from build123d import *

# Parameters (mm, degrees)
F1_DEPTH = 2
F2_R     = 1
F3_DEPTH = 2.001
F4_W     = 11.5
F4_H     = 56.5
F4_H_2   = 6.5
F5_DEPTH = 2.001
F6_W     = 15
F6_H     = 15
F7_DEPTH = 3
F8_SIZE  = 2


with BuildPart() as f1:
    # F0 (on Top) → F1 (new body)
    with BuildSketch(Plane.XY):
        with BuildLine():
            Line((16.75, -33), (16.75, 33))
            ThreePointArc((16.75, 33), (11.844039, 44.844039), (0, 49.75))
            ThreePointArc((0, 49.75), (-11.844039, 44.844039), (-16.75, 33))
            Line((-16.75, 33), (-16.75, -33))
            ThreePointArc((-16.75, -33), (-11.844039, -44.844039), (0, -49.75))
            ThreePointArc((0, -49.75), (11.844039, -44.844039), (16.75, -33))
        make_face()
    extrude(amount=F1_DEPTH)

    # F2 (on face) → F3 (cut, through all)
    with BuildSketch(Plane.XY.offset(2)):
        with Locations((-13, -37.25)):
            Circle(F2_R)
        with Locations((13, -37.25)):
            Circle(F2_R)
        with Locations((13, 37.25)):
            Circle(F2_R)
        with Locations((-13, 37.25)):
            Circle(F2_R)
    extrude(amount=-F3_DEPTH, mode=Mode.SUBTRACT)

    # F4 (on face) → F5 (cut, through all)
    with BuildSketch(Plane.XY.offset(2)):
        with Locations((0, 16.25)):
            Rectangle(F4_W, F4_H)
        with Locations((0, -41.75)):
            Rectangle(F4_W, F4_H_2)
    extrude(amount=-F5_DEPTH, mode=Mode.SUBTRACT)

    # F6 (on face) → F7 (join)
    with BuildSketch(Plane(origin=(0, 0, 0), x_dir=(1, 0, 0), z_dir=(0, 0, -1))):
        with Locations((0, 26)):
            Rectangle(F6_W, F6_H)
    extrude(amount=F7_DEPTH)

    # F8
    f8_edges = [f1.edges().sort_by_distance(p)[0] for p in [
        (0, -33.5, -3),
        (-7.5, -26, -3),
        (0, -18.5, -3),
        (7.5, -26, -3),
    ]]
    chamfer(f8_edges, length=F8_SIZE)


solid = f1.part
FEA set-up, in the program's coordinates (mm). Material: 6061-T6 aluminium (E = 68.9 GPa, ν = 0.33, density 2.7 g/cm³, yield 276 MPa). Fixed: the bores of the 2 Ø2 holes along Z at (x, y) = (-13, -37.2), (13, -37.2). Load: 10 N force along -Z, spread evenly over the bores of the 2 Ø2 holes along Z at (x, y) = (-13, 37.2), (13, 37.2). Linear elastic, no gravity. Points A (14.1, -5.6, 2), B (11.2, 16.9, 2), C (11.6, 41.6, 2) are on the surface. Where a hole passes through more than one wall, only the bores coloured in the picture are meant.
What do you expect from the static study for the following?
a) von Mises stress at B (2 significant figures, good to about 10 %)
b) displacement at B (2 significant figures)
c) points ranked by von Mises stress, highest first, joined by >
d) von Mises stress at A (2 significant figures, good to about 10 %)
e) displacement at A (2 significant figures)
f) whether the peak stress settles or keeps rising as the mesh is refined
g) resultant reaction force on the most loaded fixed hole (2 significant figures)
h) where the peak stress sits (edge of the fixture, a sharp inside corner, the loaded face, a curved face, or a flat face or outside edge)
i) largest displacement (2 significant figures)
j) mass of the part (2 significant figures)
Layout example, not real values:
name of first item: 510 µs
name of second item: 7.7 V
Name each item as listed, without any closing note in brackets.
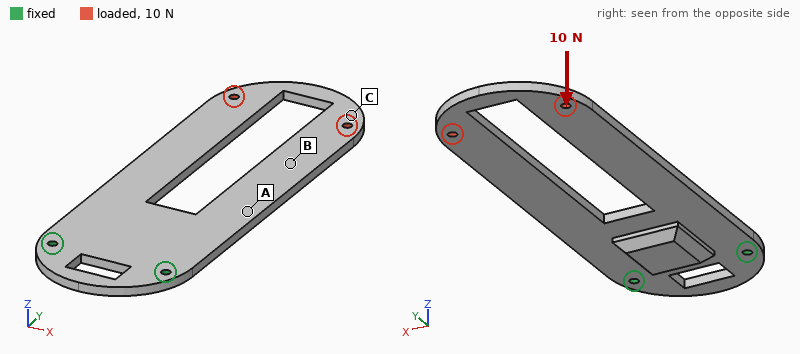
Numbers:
von Mises stress at B: 14 MPa
displacement at B: 0.51 mm
points ranked by von Mises stress, highest first, joined by >: A > B > C
von Mises stress at A: 29 MPa
displacement at A: 0.18 mm
whether the peak stress settles or keeps rising as the mesh is refined: keeps rising
resultant reaction force on the most loaded fixed hole: 5.3 N
where the peak stress sits: edge of the fixture
largest displacement: 1.2 mm
mass of the part: 14 g
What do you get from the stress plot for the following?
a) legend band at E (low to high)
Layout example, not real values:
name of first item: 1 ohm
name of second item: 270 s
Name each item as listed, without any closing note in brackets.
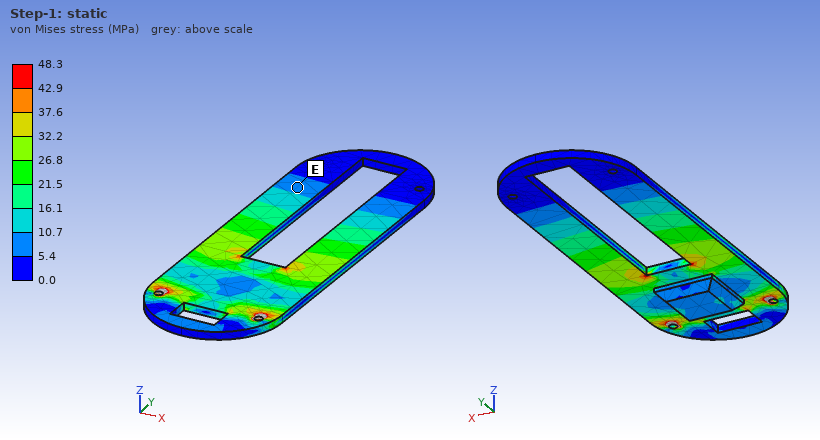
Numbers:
legend band at E: 5.4 to 10.7 MPa
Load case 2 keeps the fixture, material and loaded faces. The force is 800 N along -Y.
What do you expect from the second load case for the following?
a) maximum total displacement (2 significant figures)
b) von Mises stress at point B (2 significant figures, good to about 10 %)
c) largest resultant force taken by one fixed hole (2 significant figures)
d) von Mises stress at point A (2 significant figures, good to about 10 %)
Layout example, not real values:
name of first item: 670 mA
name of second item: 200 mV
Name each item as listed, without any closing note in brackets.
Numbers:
maximum total displacement: 32 µm
von Mises stress at point B: 18 MPa
largest resultant force taken by one fixed hole: 400 N
von Mises stress at point A: 15 MPa
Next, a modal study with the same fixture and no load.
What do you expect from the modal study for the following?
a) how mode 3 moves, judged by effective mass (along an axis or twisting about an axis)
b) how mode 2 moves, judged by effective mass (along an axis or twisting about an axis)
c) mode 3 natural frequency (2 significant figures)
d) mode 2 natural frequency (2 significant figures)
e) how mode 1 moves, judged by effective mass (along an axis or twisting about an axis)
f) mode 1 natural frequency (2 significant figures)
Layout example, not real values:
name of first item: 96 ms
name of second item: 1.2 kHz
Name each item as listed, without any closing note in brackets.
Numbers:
how mode 3 moves, judged by effective mass: along Z
how mode 2 moves, judged by effective mass: twisting about Y
mode 3 natural frequency: 1400 Hz
mode 2 natural frequency: 1100 Hz
how mode 1 moves, judged by effective mass: along Z
mode 1 natural frequency: 290 Hz
